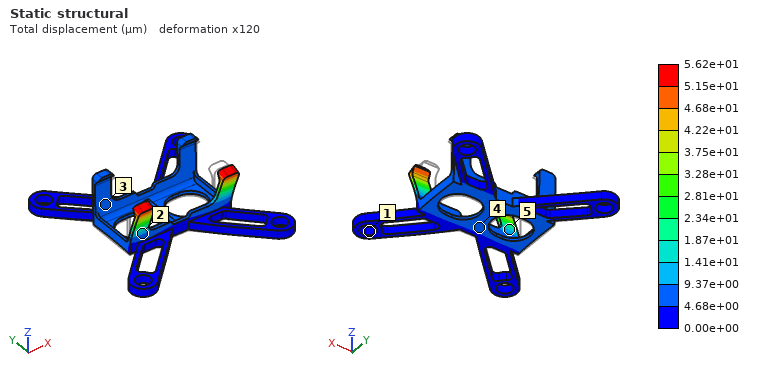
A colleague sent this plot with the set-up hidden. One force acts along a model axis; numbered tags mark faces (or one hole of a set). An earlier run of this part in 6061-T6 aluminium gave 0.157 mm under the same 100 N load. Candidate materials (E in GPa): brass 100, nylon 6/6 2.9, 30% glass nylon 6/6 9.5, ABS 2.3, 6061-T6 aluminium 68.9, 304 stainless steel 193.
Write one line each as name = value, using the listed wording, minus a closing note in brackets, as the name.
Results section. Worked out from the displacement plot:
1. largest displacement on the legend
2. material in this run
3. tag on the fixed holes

largest displacement on the legend = 5.62e+01 µm
material in this run = 304 stainless steel
tag on the fixed holes = 1
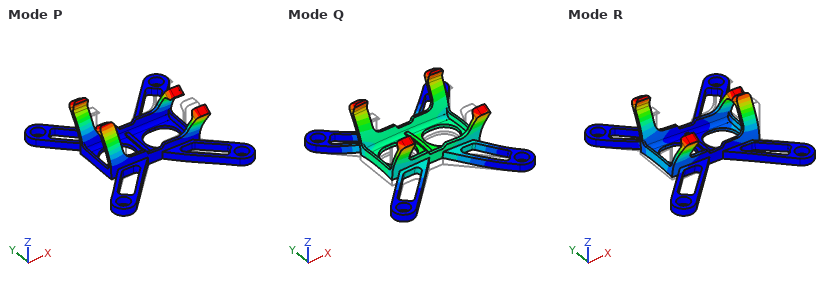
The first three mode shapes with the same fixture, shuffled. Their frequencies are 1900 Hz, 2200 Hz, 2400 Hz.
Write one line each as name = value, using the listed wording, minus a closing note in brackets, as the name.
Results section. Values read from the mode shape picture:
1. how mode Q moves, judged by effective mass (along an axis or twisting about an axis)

how mode Q moves, judged by effective mass = along Z
